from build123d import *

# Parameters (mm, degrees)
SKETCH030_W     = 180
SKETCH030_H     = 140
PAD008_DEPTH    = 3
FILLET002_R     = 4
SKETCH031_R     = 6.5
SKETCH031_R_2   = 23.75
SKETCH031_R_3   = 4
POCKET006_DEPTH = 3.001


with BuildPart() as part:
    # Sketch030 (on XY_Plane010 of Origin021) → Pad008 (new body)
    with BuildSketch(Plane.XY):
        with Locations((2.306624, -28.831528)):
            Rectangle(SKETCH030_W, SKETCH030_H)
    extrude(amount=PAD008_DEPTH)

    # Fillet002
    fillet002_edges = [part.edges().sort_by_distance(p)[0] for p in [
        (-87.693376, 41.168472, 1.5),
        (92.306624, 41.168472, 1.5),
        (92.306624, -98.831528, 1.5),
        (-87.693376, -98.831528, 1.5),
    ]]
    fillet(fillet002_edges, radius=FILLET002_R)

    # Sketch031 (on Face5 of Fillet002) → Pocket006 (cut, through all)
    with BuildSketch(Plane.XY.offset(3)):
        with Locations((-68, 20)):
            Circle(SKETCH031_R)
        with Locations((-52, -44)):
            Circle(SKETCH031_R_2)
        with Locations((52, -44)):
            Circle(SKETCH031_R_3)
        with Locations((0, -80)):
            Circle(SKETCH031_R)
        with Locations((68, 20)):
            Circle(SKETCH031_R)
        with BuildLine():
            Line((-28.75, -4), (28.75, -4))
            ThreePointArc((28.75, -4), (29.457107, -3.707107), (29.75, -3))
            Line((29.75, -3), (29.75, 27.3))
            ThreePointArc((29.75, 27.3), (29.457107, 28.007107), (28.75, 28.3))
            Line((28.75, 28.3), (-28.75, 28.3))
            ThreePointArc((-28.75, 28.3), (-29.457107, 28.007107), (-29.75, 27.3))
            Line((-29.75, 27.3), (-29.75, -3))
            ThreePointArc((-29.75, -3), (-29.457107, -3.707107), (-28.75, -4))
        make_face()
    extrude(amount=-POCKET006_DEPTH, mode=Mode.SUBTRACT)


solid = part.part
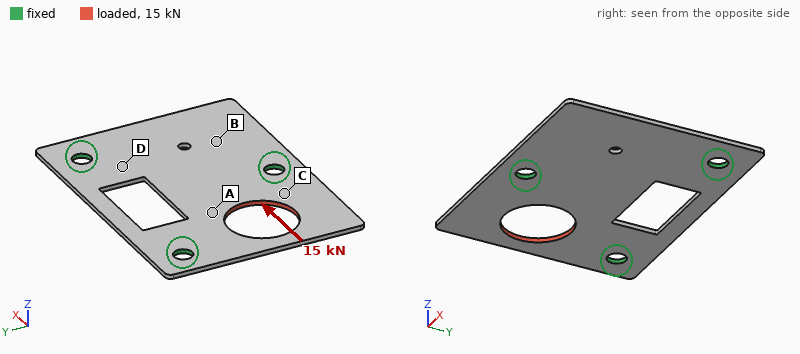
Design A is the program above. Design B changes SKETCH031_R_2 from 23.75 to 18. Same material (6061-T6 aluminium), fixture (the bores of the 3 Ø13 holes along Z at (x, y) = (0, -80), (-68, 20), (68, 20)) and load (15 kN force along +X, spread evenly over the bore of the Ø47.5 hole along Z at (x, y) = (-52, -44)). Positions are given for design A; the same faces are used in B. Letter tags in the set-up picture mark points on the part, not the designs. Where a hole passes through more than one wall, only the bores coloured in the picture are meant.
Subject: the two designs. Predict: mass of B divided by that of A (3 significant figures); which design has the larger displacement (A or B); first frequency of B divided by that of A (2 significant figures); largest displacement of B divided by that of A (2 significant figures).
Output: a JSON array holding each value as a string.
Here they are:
["1.04", "A", "1.0", "0.77"]
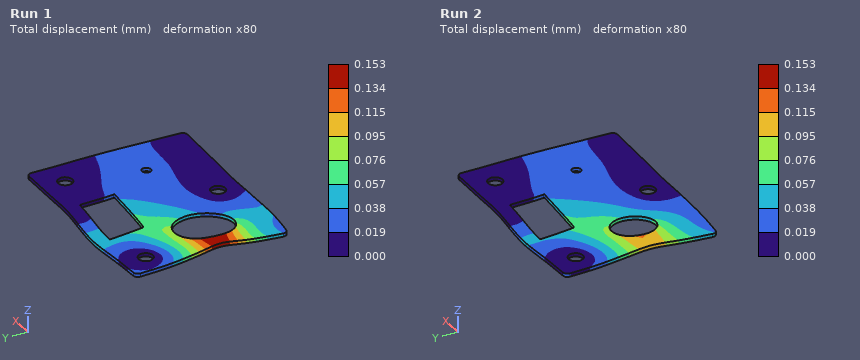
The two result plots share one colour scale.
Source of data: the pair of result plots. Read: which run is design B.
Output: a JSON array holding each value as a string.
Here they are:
["Run 2"]
